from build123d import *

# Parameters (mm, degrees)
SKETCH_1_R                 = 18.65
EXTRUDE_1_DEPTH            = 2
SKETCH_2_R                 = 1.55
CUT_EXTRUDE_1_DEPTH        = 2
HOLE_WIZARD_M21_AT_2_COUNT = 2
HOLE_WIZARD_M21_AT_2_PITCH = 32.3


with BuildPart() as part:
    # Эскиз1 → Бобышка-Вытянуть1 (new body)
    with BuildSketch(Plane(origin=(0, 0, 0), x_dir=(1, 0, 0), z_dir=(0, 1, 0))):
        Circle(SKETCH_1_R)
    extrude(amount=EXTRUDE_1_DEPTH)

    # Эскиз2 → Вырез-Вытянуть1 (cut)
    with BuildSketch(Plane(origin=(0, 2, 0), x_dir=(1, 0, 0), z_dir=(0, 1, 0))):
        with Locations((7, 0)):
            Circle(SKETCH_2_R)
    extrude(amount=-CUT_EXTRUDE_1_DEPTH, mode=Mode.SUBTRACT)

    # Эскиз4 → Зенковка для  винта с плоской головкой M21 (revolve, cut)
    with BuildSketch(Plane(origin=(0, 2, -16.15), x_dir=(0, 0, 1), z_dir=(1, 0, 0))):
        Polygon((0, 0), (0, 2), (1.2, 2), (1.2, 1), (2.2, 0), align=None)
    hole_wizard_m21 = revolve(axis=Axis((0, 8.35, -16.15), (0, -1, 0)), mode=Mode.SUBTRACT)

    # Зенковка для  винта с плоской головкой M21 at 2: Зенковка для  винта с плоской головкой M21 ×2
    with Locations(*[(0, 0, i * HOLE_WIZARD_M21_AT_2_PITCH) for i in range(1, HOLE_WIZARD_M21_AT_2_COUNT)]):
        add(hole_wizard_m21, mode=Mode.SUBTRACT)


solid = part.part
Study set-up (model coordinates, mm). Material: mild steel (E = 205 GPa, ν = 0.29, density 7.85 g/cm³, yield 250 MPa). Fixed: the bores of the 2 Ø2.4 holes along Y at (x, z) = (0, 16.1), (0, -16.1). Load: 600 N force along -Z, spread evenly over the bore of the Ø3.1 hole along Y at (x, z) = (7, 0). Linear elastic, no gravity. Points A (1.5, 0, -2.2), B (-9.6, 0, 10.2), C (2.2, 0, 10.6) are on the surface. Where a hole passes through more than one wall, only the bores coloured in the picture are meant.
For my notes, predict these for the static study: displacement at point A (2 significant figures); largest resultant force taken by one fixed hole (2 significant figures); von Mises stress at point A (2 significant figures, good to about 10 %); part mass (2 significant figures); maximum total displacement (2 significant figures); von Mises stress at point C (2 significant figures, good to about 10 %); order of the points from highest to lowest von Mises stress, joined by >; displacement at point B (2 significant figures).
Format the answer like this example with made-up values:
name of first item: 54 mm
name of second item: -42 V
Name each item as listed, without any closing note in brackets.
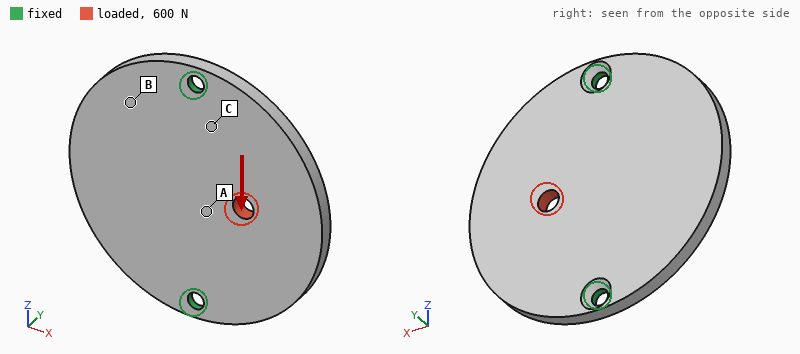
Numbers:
displacement at point A: 1.1 µm
largest resultant force taken by one fixed hole: 330 N
von Mises stress at point A: 13 MPa
part mass: 17 g
maximum total displacement: 2.2 µm
von Mises stress at point C: 22 MPa
order of the points from highest to lowest von Mises stress, joined by >: C > A > B
displacement at point B: 0.56 µm
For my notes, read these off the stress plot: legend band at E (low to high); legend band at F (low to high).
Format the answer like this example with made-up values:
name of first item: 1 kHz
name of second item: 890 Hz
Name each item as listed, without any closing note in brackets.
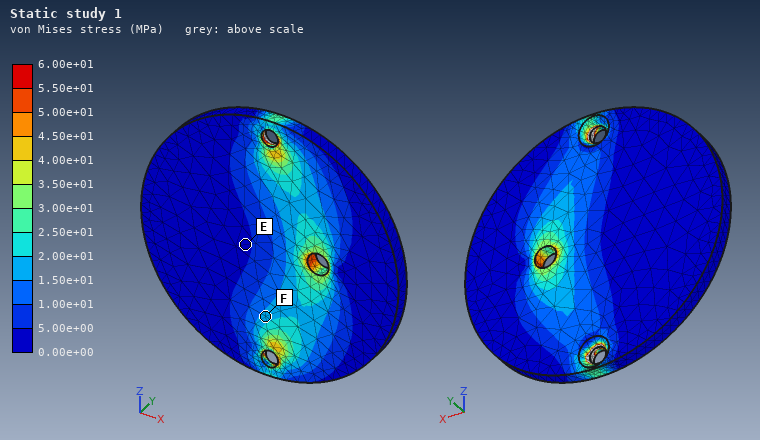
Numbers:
legend band at E: 0.00e+00 to 5.00e+00 MPa
legend band at F: 1.50e+01 to 2.00e+01 MPa
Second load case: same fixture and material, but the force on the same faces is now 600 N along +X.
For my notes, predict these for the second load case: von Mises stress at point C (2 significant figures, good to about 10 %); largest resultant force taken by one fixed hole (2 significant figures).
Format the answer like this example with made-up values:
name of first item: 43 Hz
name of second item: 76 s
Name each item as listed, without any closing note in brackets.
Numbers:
von Mises stress at point C: 11 MPa
largest resultant force taken by one fixed hole: 300 N
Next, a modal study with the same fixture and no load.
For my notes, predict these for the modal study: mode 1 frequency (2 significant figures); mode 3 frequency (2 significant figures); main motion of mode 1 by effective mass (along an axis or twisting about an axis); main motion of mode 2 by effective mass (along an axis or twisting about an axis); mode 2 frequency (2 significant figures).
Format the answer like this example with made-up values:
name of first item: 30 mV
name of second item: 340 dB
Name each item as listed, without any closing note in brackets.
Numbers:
mode 1 frequency: 3000 Hz
mode 3 frequency: 10 kHz
main motion of mode 1 by effective mass: twisting about Z
main motion of mode 2 by effective mass: along Y
mode 2 frequency: 4600 Hz
